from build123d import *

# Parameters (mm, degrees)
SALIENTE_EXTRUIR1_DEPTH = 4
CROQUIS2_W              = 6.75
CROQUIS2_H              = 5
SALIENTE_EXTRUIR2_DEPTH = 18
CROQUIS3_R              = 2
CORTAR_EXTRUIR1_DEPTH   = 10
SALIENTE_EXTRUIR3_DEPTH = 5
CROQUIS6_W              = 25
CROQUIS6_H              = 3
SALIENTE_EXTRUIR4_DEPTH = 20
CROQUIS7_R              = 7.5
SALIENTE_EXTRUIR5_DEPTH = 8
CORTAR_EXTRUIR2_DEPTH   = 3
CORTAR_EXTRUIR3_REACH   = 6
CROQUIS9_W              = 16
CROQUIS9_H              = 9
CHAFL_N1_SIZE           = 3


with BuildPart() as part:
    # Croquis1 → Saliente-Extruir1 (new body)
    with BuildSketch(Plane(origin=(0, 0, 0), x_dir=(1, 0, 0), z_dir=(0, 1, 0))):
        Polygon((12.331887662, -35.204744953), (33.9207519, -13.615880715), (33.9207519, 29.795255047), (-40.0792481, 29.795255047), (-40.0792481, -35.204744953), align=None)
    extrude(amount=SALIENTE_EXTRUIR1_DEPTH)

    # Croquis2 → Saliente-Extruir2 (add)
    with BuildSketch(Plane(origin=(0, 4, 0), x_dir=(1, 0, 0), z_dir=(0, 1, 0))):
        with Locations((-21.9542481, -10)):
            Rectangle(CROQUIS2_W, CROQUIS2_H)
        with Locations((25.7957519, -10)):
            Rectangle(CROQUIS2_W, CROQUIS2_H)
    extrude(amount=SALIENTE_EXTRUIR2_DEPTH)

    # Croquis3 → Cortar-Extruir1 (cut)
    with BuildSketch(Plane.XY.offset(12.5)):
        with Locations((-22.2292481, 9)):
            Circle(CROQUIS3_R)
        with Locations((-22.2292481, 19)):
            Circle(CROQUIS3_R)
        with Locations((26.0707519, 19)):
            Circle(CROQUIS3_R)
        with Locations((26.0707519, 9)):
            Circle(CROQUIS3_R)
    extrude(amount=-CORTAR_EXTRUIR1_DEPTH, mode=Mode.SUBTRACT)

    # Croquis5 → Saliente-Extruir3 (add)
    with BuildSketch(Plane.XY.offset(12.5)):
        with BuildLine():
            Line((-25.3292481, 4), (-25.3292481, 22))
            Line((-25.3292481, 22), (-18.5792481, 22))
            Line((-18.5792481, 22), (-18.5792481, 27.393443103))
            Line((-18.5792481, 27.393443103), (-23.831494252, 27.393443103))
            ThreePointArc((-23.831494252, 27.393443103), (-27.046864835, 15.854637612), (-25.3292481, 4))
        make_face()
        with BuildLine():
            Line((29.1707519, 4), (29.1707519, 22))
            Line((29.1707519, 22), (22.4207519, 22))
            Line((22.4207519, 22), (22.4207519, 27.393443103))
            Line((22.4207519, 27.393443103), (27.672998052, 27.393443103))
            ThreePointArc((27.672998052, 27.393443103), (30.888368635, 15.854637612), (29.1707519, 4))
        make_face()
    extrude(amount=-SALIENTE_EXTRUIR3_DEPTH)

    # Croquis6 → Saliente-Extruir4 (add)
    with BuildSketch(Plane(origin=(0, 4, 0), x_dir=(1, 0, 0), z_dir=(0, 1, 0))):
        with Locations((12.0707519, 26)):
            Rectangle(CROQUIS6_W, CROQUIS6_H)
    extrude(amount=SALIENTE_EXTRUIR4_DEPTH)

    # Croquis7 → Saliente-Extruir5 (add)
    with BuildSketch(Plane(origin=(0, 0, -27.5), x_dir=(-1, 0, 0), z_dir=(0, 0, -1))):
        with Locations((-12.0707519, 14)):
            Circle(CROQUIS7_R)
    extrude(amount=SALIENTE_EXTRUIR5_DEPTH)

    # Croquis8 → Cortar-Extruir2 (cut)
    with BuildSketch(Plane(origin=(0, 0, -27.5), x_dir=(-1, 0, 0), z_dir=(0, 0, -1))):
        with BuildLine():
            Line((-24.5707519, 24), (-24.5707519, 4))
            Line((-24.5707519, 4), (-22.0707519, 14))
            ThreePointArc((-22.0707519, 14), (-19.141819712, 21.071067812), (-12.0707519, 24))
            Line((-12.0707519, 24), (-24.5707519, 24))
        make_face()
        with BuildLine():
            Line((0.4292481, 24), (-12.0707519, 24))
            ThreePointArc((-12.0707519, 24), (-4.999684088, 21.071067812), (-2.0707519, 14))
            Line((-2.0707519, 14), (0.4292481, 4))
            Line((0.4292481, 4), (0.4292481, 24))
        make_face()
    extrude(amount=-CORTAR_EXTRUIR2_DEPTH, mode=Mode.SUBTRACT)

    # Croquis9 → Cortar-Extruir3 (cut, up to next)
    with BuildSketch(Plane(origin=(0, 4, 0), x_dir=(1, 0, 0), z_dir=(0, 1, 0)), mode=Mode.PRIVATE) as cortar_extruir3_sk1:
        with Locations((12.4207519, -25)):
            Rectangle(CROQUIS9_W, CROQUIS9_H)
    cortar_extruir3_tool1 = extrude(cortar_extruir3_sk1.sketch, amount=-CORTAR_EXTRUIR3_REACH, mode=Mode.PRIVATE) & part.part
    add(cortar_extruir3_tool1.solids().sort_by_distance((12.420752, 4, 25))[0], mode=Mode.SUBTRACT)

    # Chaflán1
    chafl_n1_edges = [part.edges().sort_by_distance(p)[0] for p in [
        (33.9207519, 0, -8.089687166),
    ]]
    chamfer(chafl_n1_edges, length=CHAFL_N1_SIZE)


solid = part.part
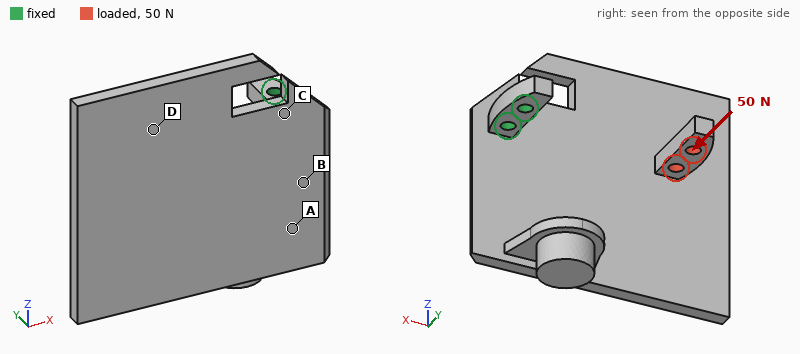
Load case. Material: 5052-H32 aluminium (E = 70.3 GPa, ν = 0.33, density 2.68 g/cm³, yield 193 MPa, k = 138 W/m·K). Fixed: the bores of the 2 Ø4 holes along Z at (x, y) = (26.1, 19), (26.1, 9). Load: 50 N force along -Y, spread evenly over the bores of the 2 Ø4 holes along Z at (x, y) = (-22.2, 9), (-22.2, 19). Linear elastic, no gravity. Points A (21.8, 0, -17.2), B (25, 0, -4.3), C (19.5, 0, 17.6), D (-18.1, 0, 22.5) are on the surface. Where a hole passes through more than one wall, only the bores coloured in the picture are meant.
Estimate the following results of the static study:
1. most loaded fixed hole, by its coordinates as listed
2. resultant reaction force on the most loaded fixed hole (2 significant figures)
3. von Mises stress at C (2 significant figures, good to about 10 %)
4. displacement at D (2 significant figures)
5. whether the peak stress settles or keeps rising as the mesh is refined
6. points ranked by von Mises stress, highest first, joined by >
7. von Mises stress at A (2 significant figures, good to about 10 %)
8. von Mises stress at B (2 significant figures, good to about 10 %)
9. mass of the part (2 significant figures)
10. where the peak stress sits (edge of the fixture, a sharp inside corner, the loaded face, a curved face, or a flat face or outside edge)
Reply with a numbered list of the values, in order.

1. (26.1, 9)
2. 89 N
3. 25 MPa
4. 0.18 mm
5. keeps rising
6. C > B > A > D
7. 7.7 MPa
8. 15 MPa
9. 58 g
10. a sharp inside corner
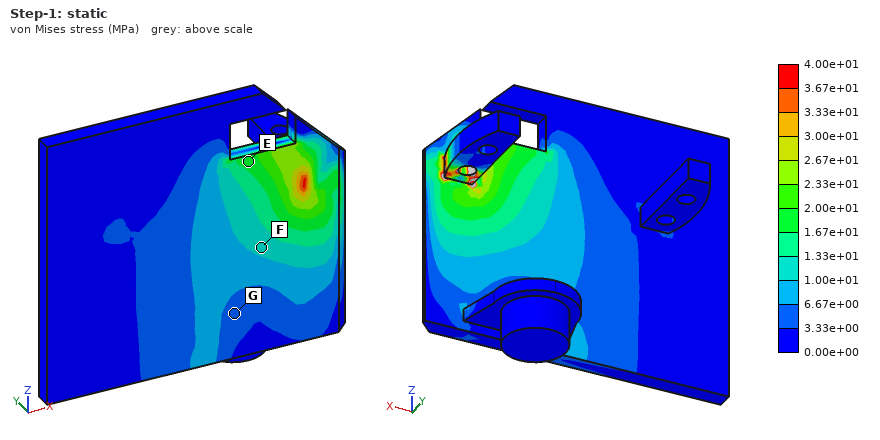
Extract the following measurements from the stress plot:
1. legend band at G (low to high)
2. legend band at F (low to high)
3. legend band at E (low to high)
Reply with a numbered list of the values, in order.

1. 3.33e+00 to 6.67e+00 MPa
2. 1.00e+01 to 1.33e+01 MPa
3. 1.67e+01 to 2.00e+01 MPa
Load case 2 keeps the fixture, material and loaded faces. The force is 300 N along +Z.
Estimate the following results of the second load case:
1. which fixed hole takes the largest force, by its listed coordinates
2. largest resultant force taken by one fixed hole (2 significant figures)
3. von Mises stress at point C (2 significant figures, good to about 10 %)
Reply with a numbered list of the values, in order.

1. (26.1, 9)
2. 280 N
3. 43 MPa
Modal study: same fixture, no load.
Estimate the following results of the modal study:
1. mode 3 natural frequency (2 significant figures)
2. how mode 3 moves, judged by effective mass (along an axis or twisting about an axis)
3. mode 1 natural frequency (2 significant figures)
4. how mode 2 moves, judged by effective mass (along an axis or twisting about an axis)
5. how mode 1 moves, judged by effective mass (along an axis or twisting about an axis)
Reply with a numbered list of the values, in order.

1. 660 Hz
2. twisting about X
3. 430 Hz
4. along Z
5. along Y
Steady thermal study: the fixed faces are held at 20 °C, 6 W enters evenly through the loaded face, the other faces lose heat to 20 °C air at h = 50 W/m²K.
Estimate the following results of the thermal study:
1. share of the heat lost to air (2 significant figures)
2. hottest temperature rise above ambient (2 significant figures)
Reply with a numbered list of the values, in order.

1. 64 %
2. 25 K
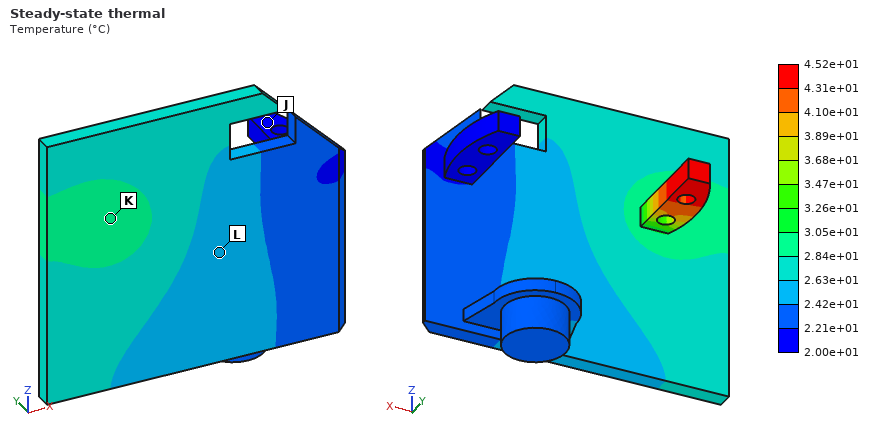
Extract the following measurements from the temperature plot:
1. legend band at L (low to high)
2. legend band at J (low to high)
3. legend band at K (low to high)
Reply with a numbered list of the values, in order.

1. 2.42e+01 to 2.63e+01 °C
2. 2.00e+01 to 2.21e+01 °C
3. 2.84e+01 to 3.05e+01 °C
